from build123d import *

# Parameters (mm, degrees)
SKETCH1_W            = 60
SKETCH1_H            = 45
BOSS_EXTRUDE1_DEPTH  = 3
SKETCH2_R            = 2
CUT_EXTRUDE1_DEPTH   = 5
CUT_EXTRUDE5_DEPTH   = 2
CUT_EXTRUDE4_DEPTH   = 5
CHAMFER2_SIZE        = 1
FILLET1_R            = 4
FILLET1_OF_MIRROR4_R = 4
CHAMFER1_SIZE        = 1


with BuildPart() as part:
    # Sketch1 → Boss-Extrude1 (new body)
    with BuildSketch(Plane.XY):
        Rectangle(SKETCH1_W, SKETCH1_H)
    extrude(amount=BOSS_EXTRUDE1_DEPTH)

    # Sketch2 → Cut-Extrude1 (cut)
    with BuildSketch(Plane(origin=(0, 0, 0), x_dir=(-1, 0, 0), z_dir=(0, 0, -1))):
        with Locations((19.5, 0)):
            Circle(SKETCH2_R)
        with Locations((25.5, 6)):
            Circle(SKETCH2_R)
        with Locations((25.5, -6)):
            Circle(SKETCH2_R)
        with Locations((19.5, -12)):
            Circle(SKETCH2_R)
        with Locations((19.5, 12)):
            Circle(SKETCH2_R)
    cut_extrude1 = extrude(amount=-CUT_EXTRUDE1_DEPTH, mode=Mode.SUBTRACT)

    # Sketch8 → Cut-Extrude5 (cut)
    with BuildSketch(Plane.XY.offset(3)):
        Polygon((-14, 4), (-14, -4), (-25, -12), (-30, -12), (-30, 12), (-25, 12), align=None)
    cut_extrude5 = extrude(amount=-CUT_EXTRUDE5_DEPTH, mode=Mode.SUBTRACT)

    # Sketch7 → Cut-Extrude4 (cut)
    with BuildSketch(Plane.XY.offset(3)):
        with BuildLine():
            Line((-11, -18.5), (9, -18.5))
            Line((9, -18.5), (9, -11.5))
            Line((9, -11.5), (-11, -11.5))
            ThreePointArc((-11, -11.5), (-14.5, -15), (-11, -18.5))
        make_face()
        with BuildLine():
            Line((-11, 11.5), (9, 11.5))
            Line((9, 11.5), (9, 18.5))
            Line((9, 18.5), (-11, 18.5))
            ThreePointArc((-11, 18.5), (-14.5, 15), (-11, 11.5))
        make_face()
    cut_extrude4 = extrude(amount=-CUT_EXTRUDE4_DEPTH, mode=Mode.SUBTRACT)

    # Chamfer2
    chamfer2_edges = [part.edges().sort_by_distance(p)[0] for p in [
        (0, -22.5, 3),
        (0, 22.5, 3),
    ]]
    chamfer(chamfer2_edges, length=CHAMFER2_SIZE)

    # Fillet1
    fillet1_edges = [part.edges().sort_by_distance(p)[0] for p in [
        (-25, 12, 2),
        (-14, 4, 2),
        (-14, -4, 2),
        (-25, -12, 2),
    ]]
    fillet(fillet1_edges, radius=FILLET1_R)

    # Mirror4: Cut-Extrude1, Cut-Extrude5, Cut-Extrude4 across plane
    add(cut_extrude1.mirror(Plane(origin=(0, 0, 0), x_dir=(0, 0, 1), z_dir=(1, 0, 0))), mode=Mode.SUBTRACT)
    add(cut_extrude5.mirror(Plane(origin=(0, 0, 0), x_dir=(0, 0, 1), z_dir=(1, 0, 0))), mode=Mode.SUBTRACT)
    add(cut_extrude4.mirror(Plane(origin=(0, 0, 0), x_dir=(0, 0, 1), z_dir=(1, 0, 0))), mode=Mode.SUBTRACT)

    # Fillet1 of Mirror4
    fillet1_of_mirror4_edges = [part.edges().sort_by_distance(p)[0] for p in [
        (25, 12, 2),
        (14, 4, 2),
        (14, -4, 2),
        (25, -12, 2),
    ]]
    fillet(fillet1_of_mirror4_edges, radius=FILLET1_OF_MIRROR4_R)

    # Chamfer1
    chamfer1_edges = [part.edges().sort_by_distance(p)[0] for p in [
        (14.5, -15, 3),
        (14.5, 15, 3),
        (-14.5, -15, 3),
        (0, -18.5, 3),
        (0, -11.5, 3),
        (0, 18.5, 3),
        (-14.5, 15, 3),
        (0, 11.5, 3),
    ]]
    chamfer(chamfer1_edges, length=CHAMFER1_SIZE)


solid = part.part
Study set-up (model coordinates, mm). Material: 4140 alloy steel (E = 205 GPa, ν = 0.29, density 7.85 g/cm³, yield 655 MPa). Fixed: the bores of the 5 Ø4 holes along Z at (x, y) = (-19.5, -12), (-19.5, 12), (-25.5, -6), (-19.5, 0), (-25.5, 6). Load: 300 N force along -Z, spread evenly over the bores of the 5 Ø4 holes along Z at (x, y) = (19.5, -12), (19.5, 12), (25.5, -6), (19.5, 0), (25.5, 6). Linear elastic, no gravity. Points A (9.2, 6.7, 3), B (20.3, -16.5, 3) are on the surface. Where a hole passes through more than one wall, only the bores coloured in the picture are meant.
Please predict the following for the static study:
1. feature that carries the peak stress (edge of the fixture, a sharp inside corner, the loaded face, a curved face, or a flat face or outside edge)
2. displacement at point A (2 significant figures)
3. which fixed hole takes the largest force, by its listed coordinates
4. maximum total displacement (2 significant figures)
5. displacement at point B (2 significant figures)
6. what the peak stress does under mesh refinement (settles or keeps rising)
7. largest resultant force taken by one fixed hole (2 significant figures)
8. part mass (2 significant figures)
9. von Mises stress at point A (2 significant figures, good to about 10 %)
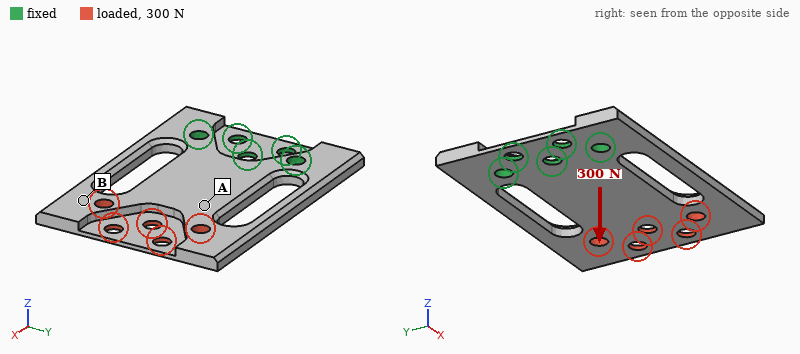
edge of the fixture
0.29 mm
(-19.5, 0)
0.70 mm
0.49 mm
keeps rising
1.1 kN
42 g
85 MPa
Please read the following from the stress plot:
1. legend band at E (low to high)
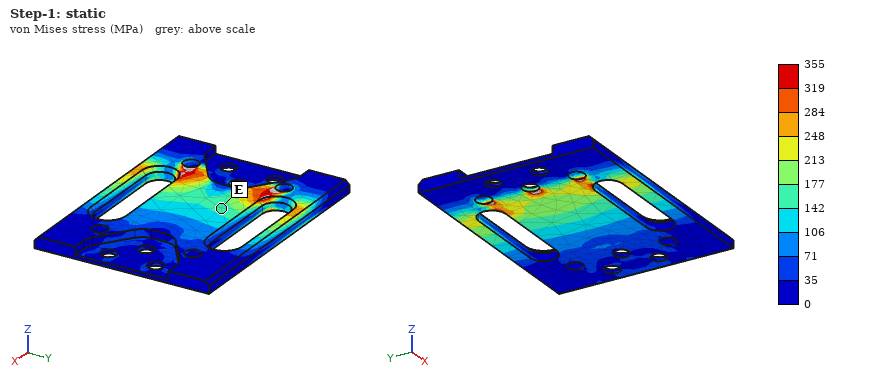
142 to 177 MPa
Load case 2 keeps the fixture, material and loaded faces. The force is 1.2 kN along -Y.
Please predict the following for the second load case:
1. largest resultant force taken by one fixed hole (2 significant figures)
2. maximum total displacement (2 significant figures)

1.9 kN
37 µm
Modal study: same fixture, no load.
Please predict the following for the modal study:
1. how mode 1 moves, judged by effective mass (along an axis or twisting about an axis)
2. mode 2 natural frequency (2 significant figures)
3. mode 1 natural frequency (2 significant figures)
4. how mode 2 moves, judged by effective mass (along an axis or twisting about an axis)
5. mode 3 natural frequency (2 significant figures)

along Z
2100 Hz
990 Hz
twisting about X
5700 Hz
